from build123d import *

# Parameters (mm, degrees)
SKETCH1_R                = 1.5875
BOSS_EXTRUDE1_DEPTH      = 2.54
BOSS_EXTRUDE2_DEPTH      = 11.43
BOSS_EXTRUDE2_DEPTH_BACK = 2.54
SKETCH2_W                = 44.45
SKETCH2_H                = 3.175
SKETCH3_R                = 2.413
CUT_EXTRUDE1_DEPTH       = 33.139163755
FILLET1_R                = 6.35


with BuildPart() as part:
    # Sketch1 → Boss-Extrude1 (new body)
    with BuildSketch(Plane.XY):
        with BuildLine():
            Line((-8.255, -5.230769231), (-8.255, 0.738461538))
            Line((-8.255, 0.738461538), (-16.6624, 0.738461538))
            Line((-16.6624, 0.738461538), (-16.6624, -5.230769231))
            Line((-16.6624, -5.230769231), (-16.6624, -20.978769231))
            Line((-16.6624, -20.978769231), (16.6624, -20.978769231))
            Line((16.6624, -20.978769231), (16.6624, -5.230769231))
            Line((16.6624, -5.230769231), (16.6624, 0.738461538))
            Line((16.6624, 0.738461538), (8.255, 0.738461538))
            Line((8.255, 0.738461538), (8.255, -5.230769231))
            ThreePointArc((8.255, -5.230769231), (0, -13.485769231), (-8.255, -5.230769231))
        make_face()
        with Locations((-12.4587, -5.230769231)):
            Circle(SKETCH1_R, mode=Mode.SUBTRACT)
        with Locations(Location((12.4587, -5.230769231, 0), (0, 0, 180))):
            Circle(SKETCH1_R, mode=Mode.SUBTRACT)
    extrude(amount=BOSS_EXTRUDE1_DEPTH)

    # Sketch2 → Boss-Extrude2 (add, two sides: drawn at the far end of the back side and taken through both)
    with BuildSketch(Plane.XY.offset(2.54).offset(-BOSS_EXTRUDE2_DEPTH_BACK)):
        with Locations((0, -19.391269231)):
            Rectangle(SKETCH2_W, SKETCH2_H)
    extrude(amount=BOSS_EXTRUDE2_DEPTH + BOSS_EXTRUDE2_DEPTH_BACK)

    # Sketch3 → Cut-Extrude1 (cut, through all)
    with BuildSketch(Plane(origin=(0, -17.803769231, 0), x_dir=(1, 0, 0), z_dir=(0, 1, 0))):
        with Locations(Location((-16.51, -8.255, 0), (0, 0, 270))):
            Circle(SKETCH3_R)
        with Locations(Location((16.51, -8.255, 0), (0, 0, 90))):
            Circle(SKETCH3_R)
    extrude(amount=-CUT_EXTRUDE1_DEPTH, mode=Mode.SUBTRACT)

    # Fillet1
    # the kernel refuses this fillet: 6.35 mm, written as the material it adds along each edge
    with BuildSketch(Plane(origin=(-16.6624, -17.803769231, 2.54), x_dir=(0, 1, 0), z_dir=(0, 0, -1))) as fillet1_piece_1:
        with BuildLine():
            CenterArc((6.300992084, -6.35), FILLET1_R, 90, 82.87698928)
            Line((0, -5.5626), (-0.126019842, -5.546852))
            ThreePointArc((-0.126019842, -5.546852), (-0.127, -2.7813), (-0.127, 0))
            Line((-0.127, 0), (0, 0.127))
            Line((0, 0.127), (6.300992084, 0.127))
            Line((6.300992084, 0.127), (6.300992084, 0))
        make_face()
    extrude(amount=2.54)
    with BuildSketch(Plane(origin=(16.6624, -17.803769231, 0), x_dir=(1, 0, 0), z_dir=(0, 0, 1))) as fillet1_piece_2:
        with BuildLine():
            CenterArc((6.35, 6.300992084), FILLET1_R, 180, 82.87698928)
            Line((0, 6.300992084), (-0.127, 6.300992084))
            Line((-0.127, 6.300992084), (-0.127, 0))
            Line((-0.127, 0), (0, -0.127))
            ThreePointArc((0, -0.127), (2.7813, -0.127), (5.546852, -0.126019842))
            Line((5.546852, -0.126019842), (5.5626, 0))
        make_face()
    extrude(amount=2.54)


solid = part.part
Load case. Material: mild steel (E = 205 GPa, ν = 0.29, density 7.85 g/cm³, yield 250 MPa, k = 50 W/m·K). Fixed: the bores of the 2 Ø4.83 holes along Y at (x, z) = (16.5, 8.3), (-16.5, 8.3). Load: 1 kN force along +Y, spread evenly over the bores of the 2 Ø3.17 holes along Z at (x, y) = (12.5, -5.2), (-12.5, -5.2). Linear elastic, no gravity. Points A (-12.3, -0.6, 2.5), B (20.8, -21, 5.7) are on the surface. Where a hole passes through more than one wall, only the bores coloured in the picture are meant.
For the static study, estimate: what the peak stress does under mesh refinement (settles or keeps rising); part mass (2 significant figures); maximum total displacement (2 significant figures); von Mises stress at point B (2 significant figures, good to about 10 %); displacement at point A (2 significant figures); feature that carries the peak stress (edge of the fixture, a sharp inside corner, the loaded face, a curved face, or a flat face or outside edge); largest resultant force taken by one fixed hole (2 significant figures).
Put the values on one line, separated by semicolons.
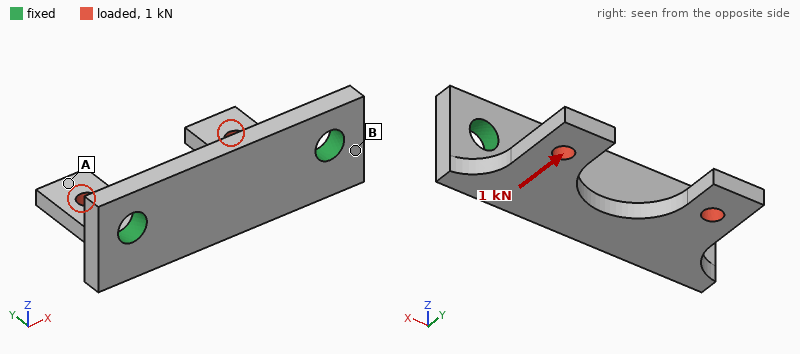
keeps rising; 23 g; 24 µm; 51 MPa; 22 µm; edge of the fixture; 510 N
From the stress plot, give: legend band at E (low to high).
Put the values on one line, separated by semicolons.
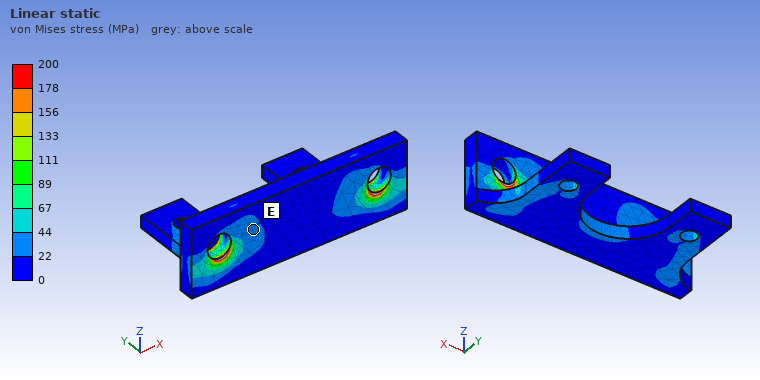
22 to 44 MPa
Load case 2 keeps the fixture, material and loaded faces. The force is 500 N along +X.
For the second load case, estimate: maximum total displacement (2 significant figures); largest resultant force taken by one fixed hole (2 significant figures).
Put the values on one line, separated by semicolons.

11 µm; 330 N
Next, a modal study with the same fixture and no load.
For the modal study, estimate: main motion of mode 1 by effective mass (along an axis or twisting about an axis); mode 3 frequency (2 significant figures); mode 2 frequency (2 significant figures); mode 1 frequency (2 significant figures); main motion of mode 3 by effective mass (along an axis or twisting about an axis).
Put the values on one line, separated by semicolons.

along Z; 14 kHz; 6300 Hz; 5700 Hz; along Y
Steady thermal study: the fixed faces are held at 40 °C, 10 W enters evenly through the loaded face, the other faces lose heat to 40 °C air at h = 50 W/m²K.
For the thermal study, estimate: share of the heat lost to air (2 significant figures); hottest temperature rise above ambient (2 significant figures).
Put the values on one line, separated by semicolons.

22 %; 60 K
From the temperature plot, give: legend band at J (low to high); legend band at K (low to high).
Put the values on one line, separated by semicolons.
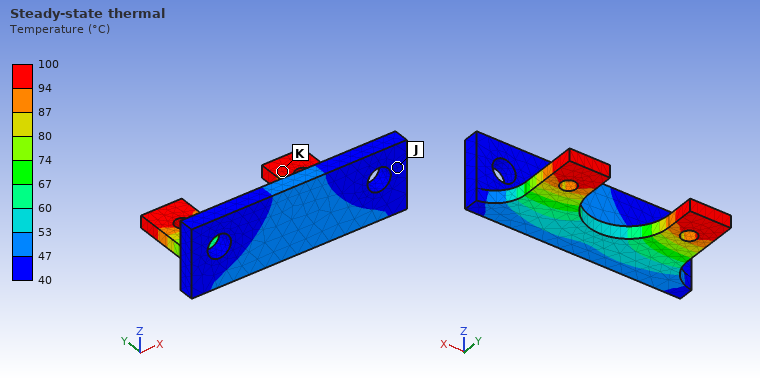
40 to 47 °C; 94 to 100 °C
